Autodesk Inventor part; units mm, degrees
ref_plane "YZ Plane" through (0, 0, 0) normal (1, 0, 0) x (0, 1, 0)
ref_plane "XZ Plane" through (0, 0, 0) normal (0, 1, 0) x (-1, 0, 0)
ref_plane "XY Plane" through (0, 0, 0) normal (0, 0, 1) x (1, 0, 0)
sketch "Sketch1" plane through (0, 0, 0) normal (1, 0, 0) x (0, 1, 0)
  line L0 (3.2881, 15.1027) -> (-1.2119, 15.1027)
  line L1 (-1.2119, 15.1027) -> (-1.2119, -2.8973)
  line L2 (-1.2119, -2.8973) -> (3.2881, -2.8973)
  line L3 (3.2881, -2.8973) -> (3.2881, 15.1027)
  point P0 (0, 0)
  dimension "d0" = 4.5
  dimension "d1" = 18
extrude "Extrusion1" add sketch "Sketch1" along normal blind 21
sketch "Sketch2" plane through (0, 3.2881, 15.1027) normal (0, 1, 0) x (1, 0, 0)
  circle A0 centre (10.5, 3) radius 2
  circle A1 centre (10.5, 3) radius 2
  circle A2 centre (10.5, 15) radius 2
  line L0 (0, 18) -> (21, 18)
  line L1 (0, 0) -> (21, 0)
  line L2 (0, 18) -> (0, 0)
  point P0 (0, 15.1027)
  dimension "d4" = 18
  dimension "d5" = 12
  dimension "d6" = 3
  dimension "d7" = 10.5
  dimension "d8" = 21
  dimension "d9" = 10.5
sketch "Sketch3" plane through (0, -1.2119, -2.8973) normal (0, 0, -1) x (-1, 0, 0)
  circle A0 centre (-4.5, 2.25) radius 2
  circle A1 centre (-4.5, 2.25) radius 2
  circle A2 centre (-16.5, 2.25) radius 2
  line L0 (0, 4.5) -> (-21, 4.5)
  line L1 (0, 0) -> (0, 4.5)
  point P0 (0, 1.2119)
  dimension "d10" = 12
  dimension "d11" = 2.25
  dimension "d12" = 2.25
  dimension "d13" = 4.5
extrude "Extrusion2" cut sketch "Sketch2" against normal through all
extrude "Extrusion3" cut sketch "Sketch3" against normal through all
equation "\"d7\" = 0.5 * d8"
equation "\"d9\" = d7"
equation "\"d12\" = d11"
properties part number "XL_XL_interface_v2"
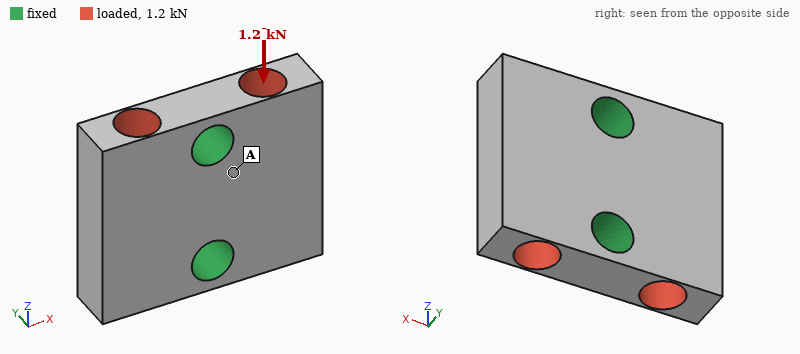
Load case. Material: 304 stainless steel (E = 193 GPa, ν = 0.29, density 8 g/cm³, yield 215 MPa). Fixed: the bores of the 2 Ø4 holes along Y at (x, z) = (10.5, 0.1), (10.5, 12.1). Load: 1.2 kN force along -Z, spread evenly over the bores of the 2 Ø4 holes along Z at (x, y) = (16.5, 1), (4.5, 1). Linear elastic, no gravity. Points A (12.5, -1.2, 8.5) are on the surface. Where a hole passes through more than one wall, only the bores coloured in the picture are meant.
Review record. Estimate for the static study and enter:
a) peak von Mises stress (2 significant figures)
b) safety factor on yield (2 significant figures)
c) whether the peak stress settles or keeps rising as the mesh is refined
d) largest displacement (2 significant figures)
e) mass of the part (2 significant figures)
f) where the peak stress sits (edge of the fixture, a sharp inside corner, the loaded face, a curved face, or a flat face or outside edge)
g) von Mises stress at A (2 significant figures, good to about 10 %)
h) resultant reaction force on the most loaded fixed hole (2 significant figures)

76 MPa
2.8
settles
1.9 µm
9.1 g
the loaded face
12 MPa
600 N
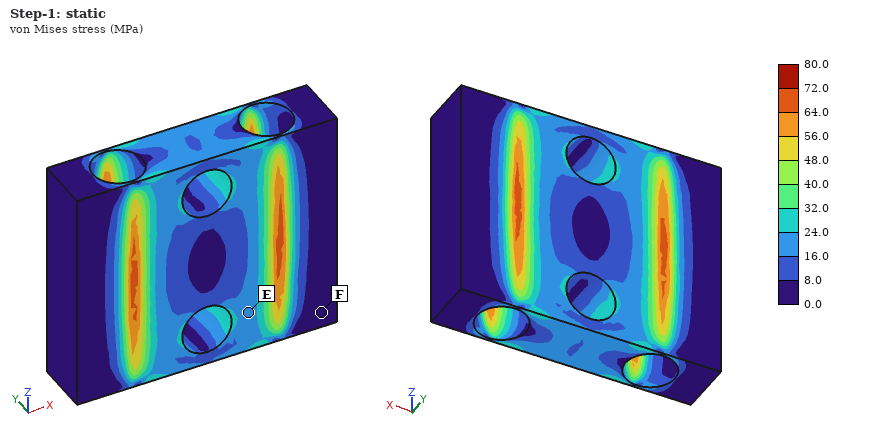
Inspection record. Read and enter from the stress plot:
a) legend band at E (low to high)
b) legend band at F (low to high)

16.0 to 24.0 MPa
0.0 to 8.0 MPa
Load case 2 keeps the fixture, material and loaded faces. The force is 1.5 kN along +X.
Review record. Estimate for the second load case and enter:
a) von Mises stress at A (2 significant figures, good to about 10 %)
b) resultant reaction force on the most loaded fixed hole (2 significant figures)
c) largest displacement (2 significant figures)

13 MPa
750 N
1.1 µm
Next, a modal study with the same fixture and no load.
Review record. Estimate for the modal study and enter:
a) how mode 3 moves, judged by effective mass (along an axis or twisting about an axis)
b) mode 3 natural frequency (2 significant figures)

twisting about X
27 kHz
